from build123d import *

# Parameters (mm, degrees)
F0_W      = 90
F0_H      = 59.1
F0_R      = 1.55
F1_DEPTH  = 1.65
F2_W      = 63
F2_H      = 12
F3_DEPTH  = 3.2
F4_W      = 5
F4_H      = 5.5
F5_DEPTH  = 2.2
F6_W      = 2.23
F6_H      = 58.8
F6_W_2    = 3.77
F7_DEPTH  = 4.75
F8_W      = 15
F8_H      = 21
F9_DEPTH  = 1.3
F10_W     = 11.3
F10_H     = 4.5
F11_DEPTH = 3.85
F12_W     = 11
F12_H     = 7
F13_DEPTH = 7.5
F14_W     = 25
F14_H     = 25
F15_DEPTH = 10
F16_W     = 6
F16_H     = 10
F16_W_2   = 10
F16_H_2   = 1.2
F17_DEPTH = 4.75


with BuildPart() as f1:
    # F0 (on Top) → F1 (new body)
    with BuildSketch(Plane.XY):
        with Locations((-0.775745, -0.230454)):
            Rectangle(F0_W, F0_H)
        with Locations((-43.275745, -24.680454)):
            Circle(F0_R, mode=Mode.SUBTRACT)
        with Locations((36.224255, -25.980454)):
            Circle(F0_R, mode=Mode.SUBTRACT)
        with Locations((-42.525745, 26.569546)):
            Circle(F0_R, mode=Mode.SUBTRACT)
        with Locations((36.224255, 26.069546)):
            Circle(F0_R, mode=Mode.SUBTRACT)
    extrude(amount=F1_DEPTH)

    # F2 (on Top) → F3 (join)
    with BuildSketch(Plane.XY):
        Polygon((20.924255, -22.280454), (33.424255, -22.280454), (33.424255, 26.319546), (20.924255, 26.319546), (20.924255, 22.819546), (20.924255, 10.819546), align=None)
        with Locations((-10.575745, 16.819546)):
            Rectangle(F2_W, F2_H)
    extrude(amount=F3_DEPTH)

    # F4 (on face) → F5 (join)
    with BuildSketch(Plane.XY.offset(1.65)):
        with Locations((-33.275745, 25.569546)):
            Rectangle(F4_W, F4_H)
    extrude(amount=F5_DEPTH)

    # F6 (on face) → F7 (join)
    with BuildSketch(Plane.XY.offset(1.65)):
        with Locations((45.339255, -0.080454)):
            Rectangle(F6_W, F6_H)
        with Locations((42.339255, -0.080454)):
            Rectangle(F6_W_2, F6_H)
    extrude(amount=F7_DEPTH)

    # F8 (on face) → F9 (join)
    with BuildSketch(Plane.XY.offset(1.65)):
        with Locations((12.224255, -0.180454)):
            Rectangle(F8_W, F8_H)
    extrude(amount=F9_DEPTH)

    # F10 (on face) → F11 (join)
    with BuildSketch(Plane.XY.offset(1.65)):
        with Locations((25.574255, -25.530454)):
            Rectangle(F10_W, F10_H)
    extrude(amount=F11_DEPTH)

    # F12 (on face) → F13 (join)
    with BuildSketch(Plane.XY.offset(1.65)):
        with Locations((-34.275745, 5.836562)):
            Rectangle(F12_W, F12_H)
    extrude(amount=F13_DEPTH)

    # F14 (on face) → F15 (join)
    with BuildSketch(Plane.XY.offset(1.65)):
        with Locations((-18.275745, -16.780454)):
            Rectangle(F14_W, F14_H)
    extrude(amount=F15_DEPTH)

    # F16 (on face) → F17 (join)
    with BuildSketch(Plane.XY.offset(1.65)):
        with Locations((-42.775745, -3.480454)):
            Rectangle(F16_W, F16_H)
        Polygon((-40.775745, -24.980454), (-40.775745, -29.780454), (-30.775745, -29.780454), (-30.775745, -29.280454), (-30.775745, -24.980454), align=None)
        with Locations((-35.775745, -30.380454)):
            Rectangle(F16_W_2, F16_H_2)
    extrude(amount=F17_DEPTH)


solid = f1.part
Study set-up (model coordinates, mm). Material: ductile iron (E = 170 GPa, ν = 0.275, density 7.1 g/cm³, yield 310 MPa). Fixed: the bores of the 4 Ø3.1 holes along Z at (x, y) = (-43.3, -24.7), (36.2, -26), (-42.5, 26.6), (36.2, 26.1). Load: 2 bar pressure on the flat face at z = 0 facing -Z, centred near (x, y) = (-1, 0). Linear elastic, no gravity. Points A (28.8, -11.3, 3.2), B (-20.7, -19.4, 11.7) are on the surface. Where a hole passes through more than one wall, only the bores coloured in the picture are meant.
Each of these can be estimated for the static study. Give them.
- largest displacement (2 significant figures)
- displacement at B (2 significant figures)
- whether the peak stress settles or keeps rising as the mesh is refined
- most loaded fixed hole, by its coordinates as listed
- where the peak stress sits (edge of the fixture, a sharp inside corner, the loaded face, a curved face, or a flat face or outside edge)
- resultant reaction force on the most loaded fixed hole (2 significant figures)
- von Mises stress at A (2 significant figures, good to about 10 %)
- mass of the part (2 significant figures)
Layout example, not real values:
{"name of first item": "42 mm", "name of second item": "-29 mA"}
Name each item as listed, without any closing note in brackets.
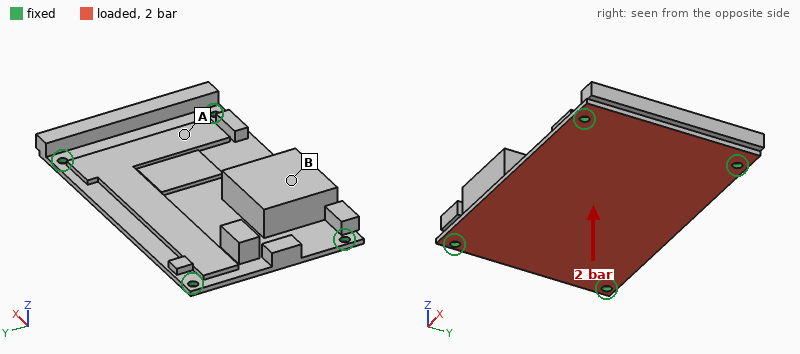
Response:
{"largest displacement": "0.25 mm", "displacement at B": "0.14 mm", "whether the peak stress settles or keeps rising as the mesh is refined": "keeps rising", "most loaded fixed hole, by its coordinates as listed": "(36.2, 26.1)", "where the peak stress sits": "edge of the fixture", "resultant reaction force on the most loaded fixed hole": "570 N", "von Mises stress at A": "53 MPa", "mass of the part": "150 g"}
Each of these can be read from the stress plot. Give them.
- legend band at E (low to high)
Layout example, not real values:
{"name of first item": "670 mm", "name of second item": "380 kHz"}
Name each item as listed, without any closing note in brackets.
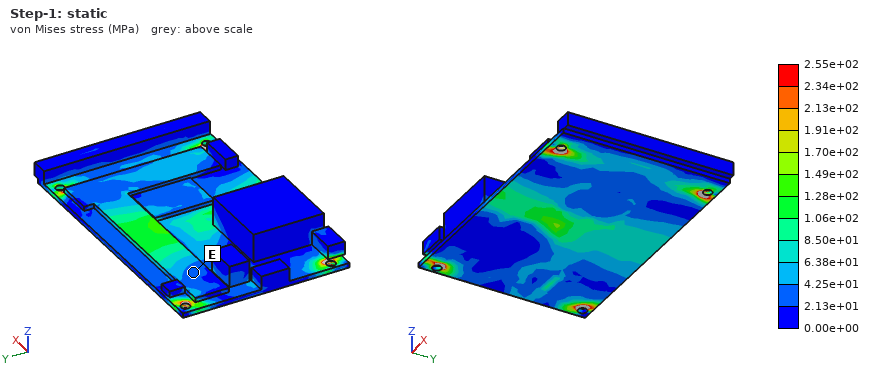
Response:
{"legend band at E": "2.13e+01 to 4.25e+01 MPa"}
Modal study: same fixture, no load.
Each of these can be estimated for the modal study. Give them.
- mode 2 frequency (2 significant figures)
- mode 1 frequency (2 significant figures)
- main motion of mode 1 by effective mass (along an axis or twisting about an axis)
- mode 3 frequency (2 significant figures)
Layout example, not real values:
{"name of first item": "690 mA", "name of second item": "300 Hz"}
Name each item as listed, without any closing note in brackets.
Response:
{"mode 2 frequency": "2000 Hz", "mode 1 frequency": "1100 Hz", "main motion of mode 1 by effective mass": "along Z", "mode 3 frequency": "3000 Hz"}
